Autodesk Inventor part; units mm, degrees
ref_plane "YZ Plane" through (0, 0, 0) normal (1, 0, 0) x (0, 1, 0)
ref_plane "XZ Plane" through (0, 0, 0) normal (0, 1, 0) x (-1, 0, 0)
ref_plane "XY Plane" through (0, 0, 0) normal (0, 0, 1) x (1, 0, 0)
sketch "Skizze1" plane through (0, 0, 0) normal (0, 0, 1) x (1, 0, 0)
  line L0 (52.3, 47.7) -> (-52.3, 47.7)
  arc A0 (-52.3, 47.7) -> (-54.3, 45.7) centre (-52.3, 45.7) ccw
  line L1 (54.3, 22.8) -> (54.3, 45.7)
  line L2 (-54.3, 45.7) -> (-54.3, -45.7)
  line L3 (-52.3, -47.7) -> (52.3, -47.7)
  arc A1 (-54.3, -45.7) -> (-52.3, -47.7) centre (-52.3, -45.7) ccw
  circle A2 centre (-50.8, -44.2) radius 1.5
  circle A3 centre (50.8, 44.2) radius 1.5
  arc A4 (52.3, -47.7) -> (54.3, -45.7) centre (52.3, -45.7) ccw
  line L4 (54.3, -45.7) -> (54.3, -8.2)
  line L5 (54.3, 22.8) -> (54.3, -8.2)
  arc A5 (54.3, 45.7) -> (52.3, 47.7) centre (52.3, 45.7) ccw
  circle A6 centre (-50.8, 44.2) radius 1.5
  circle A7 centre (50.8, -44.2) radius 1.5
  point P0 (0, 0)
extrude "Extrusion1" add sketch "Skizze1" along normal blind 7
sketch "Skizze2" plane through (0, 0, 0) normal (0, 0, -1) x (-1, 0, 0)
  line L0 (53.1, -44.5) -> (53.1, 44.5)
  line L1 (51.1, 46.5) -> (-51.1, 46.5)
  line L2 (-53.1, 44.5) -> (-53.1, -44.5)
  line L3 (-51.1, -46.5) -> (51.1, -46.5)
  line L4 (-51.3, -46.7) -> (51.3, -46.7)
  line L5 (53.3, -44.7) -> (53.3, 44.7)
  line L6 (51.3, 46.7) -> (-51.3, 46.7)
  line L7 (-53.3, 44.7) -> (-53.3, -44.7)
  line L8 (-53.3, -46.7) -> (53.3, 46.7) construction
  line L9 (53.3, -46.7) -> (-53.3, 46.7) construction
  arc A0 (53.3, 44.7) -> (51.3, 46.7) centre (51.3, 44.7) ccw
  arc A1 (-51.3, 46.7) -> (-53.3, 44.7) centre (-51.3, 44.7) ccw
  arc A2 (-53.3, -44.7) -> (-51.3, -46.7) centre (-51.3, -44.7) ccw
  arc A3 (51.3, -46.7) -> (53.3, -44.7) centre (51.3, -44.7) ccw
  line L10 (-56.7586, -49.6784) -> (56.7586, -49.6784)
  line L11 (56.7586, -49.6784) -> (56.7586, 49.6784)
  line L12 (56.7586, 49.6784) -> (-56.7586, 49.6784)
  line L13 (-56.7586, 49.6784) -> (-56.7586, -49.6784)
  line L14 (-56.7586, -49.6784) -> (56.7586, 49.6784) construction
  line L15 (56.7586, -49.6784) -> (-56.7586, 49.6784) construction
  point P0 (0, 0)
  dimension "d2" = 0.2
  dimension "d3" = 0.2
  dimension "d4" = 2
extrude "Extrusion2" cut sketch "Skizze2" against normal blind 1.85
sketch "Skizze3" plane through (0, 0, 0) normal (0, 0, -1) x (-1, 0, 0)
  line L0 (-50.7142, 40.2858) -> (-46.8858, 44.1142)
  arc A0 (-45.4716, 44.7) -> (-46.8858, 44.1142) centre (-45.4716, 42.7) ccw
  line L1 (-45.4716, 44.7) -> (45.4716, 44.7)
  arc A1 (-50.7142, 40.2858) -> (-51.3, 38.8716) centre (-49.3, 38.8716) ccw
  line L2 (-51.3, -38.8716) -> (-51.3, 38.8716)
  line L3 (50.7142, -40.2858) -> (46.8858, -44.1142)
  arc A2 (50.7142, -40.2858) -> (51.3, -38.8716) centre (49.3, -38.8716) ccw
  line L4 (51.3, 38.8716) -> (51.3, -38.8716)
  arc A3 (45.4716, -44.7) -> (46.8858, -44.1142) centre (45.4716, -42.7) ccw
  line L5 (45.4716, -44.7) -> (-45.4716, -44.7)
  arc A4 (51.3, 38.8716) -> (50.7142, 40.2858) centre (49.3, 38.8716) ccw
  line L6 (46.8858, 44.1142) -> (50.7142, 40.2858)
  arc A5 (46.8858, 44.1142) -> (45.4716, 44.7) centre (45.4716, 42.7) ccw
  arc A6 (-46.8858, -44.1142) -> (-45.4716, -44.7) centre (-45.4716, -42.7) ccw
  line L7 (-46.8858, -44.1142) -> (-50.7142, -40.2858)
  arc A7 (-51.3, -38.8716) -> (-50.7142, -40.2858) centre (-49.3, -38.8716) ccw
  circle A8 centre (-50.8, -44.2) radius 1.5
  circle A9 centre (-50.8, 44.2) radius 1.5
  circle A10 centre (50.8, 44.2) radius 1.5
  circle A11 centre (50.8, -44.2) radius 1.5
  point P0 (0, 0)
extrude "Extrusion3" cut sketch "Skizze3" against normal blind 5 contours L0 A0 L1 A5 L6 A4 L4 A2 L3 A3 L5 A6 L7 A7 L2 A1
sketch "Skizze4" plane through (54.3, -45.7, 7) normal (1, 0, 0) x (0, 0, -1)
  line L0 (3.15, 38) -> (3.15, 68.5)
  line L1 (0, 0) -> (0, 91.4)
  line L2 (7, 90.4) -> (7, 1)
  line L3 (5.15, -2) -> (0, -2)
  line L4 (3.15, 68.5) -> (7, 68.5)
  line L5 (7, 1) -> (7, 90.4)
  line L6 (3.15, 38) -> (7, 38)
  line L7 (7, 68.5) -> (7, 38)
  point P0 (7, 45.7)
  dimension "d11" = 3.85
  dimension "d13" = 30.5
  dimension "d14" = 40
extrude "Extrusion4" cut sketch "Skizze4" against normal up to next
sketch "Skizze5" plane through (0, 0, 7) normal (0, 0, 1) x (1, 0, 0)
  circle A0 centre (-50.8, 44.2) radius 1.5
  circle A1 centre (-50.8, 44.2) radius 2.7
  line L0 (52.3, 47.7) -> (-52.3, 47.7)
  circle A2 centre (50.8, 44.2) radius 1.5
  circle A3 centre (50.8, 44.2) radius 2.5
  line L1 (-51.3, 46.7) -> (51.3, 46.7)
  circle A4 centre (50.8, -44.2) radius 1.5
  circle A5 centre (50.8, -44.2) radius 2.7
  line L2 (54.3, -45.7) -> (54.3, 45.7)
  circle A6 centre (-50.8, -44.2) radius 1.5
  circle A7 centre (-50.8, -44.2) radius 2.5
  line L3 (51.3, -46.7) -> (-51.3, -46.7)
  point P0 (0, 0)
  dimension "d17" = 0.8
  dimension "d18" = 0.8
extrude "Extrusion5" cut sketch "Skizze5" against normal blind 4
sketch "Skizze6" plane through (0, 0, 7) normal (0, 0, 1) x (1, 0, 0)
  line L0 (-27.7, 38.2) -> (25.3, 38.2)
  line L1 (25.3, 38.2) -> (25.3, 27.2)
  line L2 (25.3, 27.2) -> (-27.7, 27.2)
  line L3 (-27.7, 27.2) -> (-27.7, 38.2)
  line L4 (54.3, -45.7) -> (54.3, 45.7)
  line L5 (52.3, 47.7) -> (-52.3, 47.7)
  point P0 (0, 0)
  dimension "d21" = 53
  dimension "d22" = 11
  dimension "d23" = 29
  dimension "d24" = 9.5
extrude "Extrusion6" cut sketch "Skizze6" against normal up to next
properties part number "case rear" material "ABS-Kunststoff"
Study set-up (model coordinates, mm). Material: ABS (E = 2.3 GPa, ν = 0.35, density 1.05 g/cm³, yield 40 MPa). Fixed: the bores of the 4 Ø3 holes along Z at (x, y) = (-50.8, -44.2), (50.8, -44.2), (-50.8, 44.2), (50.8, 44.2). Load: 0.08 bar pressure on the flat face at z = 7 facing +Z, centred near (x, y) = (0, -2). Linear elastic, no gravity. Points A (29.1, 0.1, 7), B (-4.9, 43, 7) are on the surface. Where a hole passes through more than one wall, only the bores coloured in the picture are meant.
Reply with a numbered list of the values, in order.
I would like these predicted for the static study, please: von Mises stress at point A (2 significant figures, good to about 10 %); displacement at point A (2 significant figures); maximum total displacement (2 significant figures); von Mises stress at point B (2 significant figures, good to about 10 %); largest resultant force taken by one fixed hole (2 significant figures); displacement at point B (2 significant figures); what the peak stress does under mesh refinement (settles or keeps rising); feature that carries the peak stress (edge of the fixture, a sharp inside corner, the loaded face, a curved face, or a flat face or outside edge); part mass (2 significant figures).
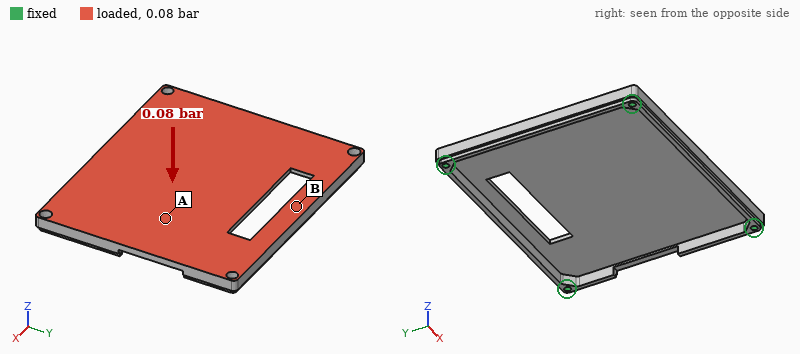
1. 3.7 MPa
2. 1.1 mm
3. 1.7 mm
4. 1.8 MPa
5. 63 N
6. 0.36 mm
7. keeps rising
8. edge of the fixture
9. 25 g
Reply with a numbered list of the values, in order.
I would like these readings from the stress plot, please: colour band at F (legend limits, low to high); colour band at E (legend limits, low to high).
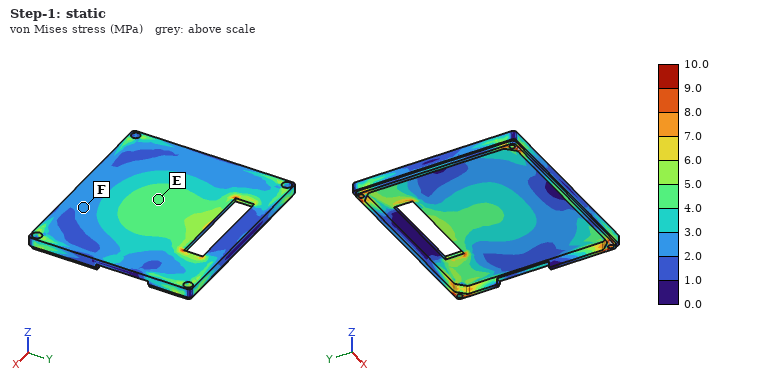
1. 2.0 to 3.0 MPa
2. 4.0 to 5.0 MPa
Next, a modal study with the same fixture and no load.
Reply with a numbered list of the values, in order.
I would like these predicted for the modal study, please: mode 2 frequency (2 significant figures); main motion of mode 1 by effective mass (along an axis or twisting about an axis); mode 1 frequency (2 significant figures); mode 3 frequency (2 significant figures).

1. 600 Hz
2. along Z
3. 290 Hz
4. 620 Hz
